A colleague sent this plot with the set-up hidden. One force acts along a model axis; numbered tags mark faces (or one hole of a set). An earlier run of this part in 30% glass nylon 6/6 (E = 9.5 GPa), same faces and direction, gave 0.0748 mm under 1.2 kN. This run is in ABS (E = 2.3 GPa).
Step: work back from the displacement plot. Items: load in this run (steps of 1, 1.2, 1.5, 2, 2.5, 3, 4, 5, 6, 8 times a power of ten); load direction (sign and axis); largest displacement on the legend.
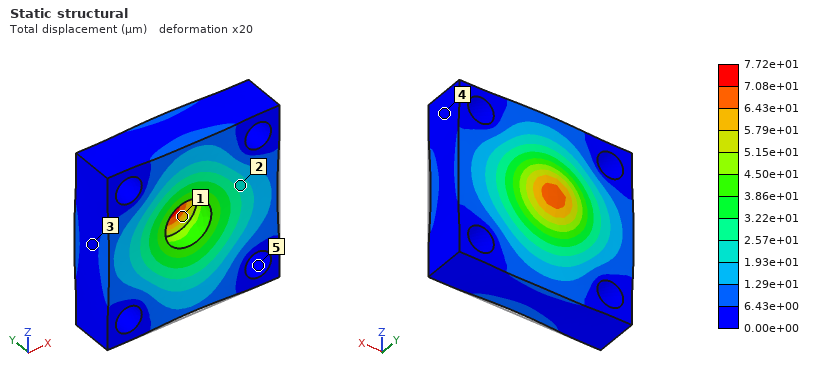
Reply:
300 N
+Y
7.72e+01 µm
